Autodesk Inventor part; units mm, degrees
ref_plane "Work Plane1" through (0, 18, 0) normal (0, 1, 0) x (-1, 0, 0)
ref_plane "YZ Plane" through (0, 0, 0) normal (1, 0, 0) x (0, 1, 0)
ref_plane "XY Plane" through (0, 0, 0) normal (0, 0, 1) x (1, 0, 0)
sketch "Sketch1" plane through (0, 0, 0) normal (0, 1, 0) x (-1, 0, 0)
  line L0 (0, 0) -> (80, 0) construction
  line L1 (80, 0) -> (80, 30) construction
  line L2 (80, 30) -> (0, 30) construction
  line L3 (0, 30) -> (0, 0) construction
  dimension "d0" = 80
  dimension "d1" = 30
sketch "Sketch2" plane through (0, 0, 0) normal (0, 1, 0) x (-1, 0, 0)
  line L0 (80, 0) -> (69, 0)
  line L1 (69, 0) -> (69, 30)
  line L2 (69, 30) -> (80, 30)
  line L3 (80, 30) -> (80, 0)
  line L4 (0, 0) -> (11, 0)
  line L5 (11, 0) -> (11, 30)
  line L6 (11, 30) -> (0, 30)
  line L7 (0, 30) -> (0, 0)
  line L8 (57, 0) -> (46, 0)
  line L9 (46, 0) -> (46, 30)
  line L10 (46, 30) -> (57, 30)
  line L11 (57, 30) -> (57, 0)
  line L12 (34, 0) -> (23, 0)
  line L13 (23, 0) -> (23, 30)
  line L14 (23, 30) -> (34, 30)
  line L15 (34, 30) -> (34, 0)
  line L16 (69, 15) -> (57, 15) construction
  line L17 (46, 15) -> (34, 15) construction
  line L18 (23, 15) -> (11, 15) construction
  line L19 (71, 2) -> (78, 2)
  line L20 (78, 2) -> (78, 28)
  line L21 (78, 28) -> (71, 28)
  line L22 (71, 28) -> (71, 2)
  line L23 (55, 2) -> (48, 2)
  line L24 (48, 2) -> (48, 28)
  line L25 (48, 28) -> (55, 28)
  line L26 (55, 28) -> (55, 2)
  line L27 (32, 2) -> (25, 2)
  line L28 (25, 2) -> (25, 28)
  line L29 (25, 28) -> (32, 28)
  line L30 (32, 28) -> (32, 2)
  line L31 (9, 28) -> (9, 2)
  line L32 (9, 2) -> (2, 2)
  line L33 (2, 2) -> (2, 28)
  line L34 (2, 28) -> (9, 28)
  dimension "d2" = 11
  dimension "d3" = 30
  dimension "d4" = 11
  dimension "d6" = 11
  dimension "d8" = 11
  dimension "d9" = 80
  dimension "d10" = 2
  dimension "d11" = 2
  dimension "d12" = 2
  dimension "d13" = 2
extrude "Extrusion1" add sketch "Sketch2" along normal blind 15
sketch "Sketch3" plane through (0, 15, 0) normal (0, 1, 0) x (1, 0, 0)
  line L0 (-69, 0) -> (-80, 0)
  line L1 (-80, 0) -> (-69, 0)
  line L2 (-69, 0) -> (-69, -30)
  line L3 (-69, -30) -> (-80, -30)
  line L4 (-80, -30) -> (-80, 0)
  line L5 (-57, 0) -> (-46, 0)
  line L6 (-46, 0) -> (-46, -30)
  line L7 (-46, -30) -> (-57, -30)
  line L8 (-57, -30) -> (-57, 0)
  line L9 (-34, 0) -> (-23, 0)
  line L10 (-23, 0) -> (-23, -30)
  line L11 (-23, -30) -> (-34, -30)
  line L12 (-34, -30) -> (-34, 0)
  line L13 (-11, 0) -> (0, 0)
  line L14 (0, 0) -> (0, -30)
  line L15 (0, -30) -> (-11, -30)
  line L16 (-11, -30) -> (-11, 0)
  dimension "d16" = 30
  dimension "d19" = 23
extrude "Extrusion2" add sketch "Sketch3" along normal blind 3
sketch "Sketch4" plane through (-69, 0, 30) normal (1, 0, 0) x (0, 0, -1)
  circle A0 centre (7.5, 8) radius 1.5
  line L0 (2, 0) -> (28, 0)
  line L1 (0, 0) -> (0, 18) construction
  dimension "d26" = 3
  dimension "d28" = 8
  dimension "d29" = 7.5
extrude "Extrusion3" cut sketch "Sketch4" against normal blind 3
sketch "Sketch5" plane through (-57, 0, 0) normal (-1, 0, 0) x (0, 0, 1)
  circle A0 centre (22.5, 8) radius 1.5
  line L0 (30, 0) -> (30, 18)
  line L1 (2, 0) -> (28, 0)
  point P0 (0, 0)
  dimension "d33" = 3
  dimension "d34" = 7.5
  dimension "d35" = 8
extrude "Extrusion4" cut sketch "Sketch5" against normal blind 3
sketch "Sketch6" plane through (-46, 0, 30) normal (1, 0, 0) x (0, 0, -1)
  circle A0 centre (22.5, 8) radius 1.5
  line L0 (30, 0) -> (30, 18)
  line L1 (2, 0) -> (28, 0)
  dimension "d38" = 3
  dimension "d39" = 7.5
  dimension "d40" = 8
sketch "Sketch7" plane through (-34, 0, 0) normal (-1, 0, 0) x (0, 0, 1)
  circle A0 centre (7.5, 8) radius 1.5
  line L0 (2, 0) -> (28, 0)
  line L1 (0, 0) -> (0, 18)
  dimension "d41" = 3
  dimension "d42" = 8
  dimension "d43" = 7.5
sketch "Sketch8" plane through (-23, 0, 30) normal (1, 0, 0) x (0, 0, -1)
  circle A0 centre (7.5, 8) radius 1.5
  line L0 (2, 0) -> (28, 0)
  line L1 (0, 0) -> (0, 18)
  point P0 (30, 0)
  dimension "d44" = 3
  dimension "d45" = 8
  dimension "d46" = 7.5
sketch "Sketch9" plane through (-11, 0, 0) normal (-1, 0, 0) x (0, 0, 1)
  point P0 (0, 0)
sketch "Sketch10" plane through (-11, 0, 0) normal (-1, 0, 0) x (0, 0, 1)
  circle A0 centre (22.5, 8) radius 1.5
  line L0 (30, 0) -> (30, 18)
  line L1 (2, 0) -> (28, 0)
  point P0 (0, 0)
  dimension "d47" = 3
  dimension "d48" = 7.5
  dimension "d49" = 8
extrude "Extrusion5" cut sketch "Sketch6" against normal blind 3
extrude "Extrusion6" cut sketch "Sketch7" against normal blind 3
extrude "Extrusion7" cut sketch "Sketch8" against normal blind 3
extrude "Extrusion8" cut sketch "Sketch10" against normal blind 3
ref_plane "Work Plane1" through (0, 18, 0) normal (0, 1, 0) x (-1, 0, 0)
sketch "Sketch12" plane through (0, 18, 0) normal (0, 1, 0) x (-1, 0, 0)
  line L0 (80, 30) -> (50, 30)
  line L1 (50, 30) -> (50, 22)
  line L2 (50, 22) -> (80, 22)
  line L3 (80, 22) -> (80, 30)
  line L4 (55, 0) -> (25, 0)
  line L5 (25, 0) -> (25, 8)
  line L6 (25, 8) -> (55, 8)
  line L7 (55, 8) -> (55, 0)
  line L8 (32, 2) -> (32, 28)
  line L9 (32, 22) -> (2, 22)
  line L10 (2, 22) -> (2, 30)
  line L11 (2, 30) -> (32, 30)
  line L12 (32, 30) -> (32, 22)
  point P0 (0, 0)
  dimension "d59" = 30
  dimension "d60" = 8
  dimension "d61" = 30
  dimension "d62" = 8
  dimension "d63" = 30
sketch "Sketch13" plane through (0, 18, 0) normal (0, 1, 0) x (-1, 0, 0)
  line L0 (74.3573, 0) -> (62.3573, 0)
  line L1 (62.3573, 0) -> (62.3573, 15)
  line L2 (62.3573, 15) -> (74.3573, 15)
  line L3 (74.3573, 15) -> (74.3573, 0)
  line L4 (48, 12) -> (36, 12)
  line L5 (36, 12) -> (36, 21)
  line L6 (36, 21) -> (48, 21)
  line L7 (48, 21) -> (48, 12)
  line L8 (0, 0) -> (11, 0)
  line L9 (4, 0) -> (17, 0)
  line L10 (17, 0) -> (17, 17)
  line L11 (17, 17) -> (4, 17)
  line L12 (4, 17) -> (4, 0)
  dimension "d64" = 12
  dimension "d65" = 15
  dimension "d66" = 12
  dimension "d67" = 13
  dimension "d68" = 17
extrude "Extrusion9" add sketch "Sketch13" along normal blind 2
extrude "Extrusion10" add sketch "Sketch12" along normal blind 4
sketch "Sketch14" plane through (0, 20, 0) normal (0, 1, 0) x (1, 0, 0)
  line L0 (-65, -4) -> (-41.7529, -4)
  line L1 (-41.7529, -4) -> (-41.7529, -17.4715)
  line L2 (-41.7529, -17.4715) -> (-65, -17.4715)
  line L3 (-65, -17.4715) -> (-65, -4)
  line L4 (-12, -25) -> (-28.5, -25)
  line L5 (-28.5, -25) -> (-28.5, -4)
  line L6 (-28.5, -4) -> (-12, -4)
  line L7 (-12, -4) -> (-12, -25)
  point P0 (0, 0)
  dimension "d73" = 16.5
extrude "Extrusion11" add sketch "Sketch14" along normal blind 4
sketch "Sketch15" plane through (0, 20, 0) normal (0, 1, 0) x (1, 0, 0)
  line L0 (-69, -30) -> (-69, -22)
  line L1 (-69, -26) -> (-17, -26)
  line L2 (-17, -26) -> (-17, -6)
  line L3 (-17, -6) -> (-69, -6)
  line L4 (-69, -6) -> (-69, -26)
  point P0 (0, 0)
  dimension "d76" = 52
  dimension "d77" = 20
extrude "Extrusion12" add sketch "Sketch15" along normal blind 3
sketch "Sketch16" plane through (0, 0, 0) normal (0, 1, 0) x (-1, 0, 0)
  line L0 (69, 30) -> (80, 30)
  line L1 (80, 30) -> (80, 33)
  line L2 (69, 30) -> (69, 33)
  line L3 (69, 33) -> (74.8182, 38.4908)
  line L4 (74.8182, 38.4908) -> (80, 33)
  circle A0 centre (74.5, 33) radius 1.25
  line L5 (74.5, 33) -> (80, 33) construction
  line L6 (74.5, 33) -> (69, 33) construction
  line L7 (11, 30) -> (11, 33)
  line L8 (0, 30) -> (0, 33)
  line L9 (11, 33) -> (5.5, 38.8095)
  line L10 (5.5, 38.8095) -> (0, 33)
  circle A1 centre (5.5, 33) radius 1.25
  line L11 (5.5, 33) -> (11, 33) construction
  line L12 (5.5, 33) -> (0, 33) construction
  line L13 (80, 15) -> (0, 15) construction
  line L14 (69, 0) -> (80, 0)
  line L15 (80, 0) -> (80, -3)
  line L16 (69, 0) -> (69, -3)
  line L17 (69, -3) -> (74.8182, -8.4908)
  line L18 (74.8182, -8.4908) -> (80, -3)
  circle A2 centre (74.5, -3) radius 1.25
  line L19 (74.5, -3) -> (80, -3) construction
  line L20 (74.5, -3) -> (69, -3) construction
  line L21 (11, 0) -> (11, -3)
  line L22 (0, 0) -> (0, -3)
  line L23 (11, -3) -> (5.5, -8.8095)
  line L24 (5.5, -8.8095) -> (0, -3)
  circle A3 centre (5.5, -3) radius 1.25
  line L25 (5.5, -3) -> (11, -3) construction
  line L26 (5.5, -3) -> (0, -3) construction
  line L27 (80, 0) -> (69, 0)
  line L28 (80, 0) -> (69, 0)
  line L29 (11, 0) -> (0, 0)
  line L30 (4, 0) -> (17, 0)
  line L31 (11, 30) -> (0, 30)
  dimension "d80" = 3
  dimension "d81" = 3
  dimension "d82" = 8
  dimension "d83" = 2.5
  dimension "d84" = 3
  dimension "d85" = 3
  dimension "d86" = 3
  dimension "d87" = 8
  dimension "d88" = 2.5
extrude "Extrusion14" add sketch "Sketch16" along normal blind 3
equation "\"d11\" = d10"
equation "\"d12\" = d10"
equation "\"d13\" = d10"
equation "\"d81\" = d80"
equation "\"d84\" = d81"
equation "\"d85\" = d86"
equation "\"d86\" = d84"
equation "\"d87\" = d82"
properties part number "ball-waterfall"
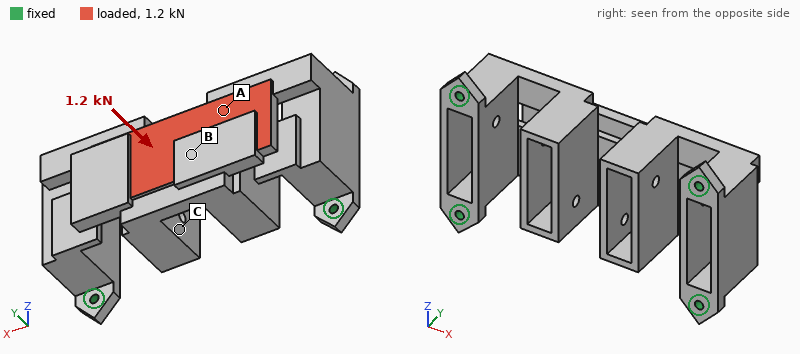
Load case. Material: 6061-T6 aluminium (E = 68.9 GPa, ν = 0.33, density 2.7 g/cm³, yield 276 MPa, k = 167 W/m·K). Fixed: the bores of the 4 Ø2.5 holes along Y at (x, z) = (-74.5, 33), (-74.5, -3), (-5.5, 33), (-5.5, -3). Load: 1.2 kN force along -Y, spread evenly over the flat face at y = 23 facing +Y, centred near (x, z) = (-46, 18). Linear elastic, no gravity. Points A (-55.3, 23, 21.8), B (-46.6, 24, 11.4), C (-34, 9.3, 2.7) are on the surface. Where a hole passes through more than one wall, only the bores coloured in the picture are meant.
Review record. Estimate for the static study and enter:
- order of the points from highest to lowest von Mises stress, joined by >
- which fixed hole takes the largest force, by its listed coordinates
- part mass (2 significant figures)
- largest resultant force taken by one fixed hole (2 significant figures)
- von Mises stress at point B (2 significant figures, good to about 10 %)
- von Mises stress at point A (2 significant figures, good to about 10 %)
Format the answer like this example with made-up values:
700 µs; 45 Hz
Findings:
B > A > C; (-74.5, 33); 57 g; 520 N; 42 MPa; 19 MPa
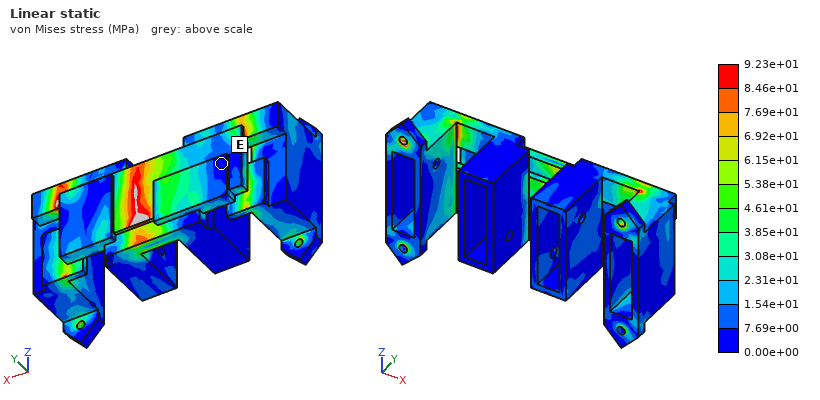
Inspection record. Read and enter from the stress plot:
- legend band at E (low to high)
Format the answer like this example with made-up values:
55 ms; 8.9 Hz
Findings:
0.00e+00 to 7.69e+00 MPa
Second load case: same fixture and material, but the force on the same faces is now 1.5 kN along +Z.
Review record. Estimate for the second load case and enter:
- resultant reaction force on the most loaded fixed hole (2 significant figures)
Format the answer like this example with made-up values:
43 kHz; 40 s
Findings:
760 N
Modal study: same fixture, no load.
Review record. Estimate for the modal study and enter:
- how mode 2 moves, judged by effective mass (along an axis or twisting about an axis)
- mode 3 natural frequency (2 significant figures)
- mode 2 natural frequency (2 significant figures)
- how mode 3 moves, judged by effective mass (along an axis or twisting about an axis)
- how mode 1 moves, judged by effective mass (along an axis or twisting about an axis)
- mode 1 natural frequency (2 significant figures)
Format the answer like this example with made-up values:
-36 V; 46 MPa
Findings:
along Y; 3800 Hz; 2700 Hz; along Z; along X; 2300 Hz
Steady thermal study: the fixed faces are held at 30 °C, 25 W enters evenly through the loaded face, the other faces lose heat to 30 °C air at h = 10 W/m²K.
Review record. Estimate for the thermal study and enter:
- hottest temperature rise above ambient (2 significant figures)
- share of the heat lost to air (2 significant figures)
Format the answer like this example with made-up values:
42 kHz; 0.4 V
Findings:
31 K; 12 %
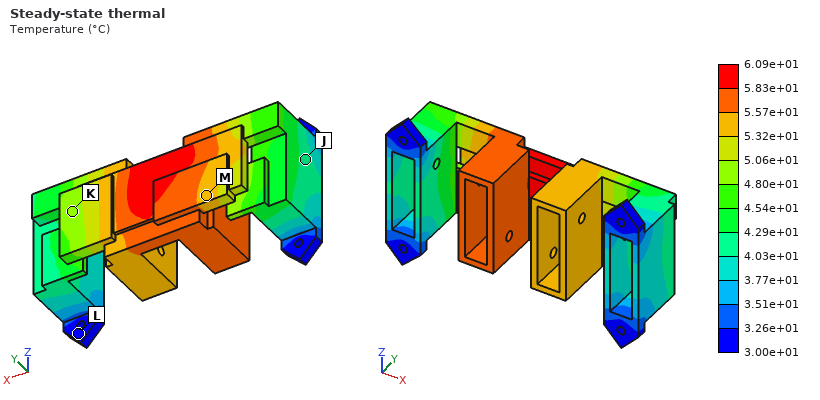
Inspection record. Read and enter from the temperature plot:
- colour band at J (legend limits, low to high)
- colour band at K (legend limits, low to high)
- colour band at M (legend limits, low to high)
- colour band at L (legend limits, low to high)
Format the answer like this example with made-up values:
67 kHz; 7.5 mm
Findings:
4.03e+01 to 4.29e+01 °C; 4.80e+01 to 5.06e+01 °C; 5.32e+01 to 5.57e+01 °C; 3.00e+01 to 3.26e+01 °C
